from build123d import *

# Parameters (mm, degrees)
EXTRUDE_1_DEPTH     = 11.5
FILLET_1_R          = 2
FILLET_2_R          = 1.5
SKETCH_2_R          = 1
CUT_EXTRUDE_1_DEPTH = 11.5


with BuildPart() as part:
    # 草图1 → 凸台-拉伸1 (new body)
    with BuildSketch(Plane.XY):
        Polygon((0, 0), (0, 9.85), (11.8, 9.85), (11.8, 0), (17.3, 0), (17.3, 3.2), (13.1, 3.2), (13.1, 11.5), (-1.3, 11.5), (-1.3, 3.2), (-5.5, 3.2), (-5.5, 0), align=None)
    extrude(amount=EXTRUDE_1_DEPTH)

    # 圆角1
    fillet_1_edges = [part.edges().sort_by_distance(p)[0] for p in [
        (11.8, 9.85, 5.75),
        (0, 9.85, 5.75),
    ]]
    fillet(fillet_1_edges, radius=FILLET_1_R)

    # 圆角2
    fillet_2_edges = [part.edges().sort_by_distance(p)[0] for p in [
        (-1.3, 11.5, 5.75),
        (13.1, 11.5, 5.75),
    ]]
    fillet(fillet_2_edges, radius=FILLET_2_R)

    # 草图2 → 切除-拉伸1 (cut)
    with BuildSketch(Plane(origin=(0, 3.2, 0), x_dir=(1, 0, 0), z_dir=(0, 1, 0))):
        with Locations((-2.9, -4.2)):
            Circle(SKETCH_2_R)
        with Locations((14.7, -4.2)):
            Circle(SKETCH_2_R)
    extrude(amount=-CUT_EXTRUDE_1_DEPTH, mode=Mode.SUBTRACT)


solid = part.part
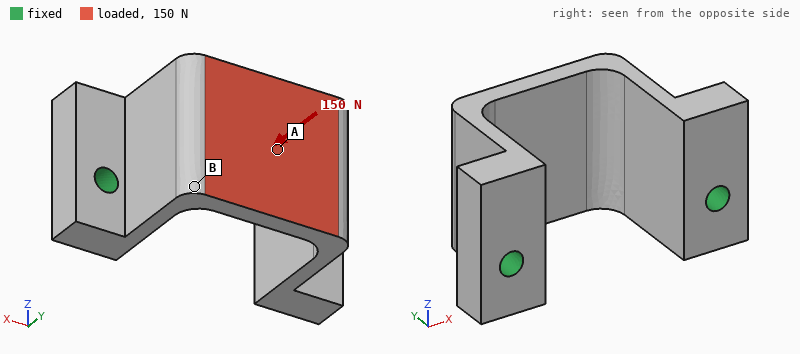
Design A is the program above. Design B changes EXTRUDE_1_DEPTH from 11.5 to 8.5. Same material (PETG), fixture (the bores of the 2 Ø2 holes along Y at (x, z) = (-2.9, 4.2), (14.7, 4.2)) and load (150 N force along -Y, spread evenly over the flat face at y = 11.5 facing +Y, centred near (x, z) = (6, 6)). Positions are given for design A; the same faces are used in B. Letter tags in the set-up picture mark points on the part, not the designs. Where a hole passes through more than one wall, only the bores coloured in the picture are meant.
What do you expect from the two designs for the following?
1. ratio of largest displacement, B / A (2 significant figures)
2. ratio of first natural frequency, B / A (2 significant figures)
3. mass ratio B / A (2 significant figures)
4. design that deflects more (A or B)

1.1
1.0
0.73
B
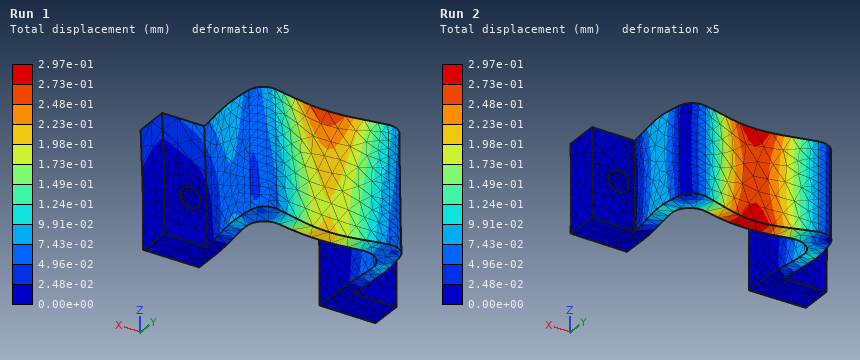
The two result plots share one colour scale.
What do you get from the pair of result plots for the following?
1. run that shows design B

Run 2
